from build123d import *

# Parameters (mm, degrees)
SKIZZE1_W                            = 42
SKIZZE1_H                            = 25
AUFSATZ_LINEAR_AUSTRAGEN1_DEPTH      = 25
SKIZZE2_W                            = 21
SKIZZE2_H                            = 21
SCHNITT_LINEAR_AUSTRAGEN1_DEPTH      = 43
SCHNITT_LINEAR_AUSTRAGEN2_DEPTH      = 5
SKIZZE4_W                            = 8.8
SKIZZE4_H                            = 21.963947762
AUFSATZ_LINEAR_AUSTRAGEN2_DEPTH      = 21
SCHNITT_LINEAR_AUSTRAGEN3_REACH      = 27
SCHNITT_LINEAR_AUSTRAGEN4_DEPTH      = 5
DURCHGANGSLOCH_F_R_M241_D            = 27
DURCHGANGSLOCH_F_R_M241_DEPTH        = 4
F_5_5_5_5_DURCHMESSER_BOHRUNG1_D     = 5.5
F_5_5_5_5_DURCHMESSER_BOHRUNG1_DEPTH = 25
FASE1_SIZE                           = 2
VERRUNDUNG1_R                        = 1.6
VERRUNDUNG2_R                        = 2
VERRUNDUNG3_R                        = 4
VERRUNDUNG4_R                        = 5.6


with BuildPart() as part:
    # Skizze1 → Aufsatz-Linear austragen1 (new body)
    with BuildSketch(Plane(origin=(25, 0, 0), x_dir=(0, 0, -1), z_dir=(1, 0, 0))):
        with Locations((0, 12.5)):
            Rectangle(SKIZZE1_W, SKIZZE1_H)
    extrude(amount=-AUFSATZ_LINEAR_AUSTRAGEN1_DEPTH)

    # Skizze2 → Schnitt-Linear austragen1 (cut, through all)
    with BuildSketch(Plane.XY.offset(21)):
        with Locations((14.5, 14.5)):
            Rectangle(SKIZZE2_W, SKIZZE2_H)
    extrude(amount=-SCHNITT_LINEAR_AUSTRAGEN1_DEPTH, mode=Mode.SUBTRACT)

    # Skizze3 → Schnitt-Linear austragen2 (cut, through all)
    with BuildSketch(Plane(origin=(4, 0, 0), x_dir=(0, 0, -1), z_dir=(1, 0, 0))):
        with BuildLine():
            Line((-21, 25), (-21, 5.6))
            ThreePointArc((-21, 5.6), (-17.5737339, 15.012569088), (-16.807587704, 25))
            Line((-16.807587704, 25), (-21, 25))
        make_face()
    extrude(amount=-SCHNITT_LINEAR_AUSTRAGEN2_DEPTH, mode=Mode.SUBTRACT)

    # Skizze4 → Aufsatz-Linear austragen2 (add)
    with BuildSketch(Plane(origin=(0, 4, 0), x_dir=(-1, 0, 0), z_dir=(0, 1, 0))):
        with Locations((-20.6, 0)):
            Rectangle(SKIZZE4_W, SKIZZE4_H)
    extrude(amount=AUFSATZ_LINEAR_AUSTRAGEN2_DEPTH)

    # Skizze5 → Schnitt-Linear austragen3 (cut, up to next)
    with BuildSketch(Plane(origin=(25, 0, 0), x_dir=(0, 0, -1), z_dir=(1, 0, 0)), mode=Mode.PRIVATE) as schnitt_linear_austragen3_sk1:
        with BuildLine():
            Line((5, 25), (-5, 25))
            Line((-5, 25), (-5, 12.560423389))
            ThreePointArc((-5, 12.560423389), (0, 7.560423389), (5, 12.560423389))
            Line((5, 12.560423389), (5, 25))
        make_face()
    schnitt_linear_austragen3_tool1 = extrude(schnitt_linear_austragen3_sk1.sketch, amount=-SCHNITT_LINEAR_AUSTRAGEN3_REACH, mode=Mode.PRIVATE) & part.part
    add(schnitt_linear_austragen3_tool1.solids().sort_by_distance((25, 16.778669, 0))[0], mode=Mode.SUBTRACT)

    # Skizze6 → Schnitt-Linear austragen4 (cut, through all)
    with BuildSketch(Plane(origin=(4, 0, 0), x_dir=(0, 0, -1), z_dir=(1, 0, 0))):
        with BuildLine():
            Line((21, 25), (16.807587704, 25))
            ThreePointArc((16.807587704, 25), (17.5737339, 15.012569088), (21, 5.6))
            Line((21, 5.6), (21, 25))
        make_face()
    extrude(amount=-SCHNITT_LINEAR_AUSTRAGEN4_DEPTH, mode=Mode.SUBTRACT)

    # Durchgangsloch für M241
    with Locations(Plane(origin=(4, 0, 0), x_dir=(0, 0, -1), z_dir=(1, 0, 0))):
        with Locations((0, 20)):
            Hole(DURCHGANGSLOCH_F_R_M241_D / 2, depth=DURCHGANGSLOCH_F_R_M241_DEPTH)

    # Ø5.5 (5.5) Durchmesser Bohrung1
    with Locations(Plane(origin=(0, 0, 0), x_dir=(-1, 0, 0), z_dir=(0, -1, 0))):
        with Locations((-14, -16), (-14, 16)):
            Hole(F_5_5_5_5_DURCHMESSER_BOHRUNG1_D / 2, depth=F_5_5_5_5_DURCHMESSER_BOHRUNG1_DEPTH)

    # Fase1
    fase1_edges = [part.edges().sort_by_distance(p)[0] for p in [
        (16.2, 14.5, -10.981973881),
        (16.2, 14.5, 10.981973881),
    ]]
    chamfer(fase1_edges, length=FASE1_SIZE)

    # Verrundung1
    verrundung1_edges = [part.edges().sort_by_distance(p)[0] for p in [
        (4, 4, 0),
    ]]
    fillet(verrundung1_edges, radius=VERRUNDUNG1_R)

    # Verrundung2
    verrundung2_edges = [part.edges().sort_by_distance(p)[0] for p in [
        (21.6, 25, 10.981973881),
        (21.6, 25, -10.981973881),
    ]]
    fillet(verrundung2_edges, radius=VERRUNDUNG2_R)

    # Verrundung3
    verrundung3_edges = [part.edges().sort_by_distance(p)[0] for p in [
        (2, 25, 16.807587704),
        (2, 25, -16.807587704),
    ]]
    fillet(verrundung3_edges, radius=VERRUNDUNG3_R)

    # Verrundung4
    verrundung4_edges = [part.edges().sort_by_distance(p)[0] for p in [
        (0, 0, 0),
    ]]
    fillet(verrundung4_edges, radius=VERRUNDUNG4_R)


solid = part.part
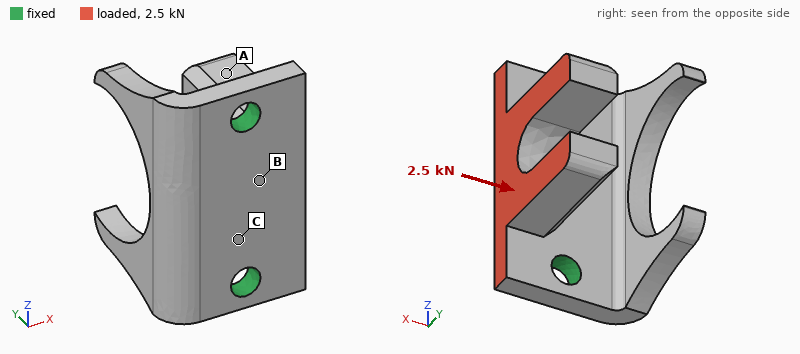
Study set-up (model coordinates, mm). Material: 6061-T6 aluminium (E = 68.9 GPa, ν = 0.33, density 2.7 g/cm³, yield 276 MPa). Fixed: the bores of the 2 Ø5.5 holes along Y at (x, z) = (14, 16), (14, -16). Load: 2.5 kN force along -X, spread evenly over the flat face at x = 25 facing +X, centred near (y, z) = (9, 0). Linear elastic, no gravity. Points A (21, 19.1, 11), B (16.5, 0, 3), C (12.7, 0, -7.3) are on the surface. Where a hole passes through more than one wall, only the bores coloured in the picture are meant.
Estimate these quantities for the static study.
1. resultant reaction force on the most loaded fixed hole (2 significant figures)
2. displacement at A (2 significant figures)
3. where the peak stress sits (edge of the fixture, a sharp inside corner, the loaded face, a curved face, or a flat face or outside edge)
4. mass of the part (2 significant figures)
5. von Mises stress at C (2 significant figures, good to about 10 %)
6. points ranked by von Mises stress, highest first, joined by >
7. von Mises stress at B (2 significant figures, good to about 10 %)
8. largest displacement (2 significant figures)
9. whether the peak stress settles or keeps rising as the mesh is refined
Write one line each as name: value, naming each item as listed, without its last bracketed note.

resultant reaction force on the most loaded fixed hole: 1.3 kN
displacement at A: 0.16 mm
where the peak stress sits: edge of the fixture
mass of the part: 21 g
von Mises stress at C: 55 MPa
points ranked by von Mises stress, highest first, joined by >: B > C > A
von Mises stress at B: 85 MPa
largest displacement: 0.22 mm
whether the peak stress settles or keeps rising as the mesh is refined: keeps rising
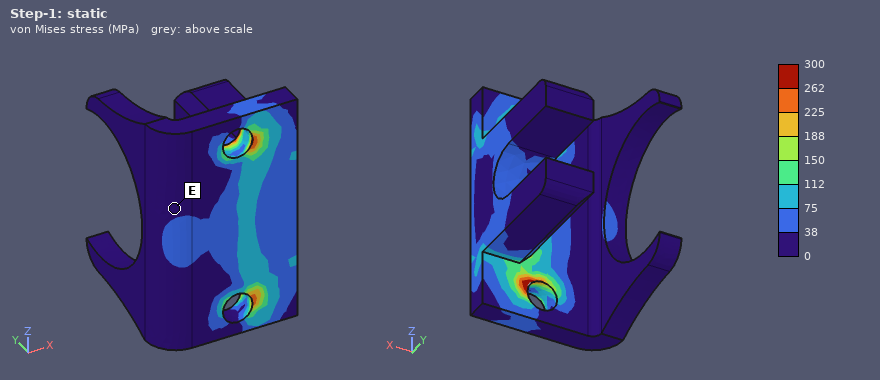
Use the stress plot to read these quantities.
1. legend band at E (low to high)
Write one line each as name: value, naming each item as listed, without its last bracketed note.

legend band at E: 0 to 38 MPa
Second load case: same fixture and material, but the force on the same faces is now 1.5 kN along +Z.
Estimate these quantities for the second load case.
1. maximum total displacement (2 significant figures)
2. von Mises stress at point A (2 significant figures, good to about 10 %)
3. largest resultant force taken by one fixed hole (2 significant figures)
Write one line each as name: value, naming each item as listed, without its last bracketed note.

maximum total displacement: 47 µm
von Mises stress at point A: 13 MPa
largest resultant force taken by one fixed hole: 980 N
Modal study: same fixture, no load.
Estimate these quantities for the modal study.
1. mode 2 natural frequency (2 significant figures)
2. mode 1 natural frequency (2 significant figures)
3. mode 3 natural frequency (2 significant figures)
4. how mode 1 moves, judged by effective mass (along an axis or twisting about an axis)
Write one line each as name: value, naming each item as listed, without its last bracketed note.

mode 2 natural frequency: 7300 Hz
mode 1 natural frequency: 5900 Hz
mode 3 natural frequency: 7900 Hz
how mode 1 moves, judged by effective mass: along X
